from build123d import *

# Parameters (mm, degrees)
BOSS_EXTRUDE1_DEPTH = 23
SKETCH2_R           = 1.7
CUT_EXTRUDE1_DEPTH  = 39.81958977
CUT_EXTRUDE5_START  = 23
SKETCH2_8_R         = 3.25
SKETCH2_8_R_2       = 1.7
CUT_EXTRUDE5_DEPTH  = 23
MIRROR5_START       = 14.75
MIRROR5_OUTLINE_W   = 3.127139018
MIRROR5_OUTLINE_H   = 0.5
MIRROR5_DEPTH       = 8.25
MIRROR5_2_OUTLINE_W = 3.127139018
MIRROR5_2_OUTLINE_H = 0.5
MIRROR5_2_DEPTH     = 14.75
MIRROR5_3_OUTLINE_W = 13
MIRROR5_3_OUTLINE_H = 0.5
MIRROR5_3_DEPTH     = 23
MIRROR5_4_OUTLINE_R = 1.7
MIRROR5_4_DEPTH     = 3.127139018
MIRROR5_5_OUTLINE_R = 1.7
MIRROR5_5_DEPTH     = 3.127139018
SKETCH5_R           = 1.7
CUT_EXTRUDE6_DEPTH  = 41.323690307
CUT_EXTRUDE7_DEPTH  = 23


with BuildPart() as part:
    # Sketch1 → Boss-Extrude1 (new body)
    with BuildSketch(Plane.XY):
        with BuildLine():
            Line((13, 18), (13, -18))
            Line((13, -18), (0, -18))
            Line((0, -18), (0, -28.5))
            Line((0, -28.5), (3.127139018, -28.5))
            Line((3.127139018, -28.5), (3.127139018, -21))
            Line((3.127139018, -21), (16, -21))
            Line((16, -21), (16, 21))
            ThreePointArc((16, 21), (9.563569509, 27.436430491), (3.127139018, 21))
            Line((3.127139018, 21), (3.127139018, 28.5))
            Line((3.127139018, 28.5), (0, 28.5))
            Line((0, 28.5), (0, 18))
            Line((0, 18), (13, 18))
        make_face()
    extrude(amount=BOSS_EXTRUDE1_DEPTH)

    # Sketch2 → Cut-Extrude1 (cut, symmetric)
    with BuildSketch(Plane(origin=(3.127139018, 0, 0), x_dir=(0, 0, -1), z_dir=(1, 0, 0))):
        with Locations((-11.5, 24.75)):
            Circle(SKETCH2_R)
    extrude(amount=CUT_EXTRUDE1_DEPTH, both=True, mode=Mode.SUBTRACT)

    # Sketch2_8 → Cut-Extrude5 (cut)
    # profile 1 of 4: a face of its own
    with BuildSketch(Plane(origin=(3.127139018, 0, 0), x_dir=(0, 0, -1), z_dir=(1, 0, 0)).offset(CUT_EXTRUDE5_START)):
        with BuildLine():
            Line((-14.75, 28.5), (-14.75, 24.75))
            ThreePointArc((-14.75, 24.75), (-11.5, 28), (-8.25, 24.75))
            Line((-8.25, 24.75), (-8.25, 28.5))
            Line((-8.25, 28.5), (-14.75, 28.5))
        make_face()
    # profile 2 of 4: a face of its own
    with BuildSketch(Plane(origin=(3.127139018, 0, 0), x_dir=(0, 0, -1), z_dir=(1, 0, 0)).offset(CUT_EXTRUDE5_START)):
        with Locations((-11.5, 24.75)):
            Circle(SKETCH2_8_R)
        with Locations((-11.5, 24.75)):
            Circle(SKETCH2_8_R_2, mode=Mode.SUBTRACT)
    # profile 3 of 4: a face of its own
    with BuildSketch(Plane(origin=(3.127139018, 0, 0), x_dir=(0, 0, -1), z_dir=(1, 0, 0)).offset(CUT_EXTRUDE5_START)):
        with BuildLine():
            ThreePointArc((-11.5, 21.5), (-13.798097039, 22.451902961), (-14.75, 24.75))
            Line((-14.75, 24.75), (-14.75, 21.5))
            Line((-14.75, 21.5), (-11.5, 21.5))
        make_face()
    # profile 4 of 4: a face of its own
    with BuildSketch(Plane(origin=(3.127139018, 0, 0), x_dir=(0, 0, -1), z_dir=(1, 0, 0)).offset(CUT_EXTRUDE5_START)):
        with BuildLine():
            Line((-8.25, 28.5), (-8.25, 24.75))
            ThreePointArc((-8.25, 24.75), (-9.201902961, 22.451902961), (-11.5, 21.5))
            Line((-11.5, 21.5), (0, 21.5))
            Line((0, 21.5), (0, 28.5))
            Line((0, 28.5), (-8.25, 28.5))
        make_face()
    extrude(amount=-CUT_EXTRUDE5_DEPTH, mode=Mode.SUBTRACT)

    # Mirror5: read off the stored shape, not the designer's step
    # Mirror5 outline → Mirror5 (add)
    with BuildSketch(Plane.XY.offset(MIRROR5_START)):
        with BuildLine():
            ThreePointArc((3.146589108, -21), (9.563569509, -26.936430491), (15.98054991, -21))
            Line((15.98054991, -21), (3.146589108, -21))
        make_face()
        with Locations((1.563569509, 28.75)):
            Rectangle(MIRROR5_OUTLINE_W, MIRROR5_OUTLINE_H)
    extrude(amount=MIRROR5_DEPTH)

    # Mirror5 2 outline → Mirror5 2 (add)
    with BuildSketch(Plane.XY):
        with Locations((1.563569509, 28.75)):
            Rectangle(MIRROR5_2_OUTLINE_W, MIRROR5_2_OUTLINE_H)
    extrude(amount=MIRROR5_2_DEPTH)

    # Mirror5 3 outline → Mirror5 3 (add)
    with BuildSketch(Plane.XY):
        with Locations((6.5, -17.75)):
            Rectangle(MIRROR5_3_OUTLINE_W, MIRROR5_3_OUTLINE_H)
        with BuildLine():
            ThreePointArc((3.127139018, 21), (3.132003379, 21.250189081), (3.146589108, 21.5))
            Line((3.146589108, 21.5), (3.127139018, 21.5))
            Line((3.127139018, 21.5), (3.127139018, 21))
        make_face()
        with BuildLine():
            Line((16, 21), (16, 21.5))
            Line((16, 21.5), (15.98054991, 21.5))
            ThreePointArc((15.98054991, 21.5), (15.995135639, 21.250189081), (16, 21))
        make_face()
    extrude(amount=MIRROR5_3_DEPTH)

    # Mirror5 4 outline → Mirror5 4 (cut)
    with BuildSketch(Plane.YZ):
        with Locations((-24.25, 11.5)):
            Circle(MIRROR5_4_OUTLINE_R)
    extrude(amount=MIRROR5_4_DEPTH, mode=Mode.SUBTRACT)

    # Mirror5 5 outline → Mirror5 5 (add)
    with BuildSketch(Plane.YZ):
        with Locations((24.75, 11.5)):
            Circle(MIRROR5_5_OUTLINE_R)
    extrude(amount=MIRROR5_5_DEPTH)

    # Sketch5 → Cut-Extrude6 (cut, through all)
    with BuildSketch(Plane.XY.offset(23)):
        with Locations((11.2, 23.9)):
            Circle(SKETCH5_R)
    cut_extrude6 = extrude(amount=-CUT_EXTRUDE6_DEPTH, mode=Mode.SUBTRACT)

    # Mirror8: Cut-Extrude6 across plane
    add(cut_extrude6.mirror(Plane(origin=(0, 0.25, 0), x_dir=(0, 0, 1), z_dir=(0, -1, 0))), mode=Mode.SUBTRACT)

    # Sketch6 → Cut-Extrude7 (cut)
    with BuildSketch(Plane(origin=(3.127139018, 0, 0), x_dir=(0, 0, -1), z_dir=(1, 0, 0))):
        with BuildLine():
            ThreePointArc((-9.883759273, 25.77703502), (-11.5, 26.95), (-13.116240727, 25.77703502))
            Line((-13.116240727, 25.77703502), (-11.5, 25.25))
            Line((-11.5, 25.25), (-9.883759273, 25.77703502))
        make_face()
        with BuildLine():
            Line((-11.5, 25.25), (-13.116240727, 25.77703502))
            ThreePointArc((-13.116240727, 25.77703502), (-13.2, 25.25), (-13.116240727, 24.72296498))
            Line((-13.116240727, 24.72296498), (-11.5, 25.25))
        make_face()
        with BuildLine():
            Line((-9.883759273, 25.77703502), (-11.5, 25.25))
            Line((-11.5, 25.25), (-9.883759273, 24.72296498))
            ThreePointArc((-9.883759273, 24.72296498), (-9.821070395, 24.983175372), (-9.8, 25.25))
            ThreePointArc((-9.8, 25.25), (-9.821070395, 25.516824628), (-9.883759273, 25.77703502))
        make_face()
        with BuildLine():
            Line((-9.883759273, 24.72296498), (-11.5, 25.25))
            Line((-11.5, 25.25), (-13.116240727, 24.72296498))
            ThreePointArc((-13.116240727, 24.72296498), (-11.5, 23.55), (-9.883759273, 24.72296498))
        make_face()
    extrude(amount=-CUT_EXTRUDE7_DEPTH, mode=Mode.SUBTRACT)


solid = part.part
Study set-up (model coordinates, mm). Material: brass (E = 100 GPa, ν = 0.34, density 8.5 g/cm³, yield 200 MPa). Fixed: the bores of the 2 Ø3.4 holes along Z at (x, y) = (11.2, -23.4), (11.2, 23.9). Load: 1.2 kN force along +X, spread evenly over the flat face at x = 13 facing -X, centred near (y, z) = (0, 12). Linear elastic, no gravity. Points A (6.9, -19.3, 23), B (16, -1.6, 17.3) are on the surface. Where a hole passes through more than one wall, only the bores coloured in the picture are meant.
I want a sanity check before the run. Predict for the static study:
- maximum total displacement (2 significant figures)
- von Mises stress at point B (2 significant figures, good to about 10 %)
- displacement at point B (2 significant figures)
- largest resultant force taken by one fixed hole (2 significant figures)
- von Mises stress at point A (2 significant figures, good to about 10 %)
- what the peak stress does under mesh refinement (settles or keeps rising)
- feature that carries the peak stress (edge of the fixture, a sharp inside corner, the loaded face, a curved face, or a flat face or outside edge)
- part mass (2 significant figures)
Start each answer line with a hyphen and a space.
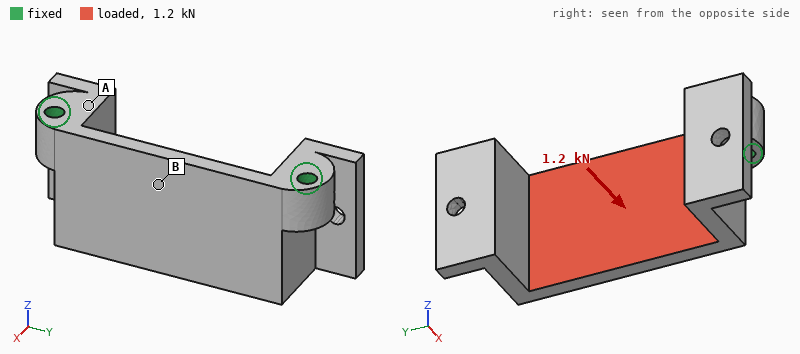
- 71 µm
- 71 MPa
- 48 µm
- 750 N
- 12 MPa
- keeps rising
- a sharp inside corner
- 58 g
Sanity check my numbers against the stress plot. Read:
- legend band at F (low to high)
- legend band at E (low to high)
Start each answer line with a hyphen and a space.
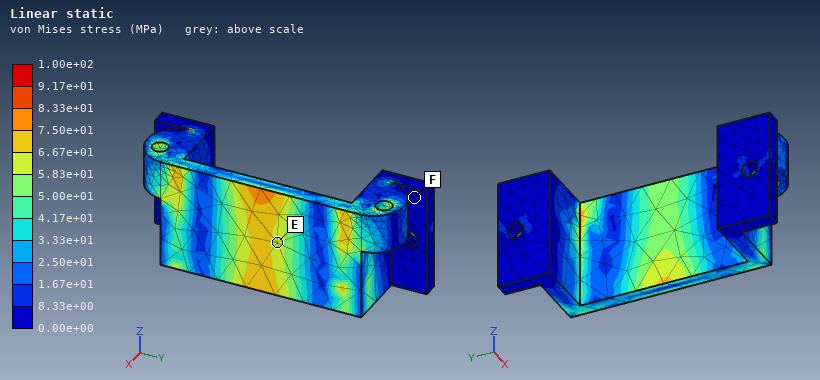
- 0.00e+00 to 8.33e+00 MPa
- 5.83e+01 to 6.67e+01 MPa
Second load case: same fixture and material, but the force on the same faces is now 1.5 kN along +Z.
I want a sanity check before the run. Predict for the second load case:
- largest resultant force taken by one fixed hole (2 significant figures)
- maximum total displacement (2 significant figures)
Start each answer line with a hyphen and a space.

- 810 N
- 14 µm
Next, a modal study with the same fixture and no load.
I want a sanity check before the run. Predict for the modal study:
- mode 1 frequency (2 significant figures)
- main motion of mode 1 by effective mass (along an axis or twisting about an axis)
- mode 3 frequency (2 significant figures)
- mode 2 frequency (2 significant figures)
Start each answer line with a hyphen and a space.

- 5300 Hz
- along X
- 7600 Hz
- 7400 Hz
